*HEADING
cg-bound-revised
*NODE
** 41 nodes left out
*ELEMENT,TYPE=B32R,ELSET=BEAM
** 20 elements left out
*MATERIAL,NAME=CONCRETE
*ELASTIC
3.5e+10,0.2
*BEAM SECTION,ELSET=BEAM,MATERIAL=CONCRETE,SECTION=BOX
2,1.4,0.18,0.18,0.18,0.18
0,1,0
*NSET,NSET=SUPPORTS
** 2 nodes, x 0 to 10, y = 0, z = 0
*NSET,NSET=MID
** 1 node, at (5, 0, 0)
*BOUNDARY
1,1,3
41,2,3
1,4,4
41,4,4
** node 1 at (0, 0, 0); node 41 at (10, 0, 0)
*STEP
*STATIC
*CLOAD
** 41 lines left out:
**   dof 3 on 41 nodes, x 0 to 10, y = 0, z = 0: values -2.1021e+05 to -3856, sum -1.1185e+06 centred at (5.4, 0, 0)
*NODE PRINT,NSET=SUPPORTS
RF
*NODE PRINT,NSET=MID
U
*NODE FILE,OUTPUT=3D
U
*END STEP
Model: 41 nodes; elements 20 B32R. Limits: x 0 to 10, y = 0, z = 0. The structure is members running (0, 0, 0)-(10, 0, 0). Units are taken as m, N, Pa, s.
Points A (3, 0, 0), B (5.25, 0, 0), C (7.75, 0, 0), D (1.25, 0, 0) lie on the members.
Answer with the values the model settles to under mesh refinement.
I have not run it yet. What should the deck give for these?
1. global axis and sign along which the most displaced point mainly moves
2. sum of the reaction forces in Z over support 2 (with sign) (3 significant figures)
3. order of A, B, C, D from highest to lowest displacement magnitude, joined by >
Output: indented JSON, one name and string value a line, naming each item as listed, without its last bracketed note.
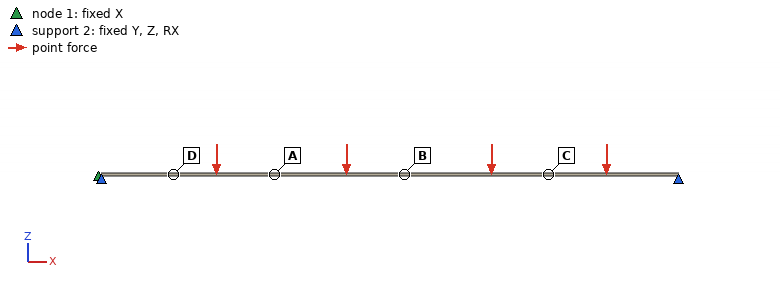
{
  "global axis and sign along which the most displaced point mainly moves": "-Z",
  "sum of the reaction forces in Z over support 2 (with sign)": "1.12e+06 N",
  "order of A, B, C, D from highest to lowest displacement magnitude, joined by >": "B > A > C > D"
}
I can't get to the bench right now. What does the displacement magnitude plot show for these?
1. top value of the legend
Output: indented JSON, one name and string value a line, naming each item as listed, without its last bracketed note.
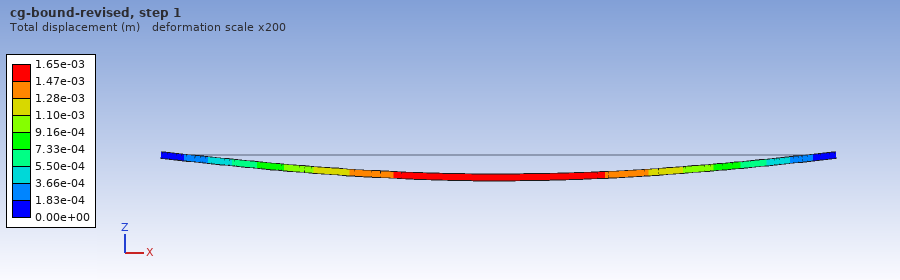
{
  "top value of the legend": "1.65e-03 m"
}
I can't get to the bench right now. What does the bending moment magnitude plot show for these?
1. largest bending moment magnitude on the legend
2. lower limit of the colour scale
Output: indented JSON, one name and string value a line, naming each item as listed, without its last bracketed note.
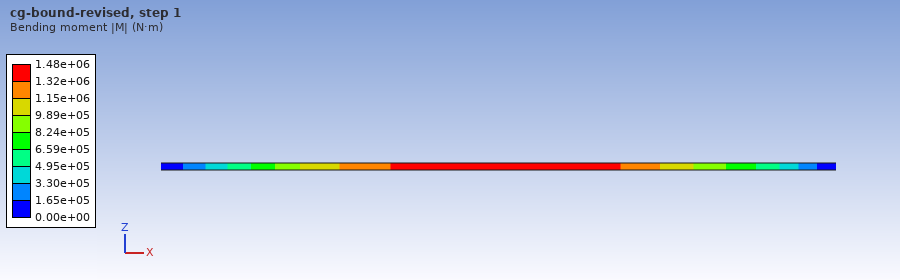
{
  "largest bending moment magnitude on the legend": "1.48e+06 N·m",
  "lower limit of the colour scale": "0.00e+00 N·m"
}
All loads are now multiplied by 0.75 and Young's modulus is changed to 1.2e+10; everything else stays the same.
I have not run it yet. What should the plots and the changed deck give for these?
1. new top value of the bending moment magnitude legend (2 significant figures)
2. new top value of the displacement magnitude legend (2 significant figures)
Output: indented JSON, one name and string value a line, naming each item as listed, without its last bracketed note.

{
  "new top value of the bending moment magnitude legend": "1.1e+06 N·m",
  "new top value of the displacement magnitude legend": "0.0036 m"
}
